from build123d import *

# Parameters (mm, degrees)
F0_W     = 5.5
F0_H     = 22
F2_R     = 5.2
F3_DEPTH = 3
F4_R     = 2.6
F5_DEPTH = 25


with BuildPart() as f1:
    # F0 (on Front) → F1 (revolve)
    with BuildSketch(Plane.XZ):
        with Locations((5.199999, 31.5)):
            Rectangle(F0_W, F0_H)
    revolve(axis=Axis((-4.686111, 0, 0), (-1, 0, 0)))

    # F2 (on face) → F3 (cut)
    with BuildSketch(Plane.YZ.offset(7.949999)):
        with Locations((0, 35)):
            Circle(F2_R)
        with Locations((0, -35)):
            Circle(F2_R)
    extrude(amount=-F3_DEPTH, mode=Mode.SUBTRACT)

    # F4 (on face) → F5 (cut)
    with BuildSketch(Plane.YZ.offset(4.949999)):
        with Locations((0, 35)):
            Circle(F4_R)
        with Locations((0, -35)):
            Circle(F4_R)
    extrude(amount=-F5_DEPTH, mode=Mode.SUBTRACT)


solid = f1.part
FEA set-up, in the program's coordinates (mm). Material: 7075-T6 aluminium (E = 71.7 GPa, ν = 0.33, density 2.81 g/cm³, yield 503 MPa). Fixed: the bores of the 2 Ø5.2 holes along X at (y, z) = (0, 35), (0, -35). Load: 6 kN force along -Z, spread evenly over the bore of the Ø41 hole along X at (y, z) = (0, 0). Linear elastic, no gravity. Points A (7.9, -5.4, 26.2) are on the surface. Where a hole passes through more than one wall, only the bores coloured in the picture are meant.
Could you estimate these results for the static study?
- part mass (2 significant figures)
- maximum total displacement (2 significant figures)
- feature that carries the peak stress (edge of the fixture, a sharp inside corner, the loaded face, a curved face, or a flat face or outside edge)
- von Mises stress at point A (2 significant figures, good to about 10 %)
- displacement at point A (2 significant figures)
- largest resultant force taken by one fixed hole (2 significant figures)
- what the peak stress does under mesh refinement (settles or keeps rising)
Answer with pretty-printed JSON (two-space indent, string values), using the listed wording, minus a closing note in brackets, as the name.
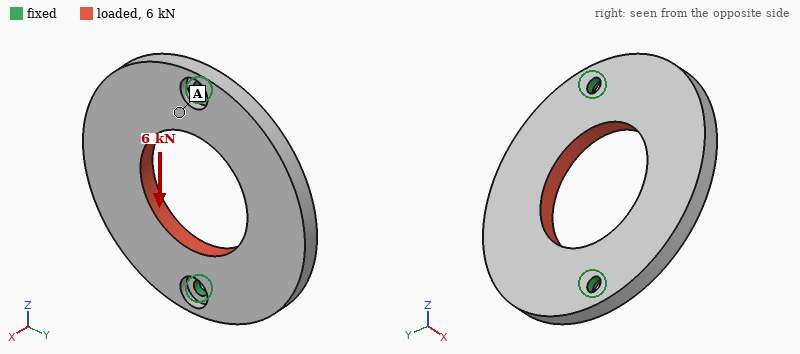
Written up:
{
  "part mass": "66 g",
  "maximum total displacement": "21 µm",
  "feature that carries the peak stress": "edge of the fixture",
  "von Mises stress at point A": "17 MPa",
  "displacement at point A": "13 µm",
  "largest resultant force taken by one fixed hole": "3.0 kN",
  "what the peak stress does under mesh refinement": "keeps rising"
}
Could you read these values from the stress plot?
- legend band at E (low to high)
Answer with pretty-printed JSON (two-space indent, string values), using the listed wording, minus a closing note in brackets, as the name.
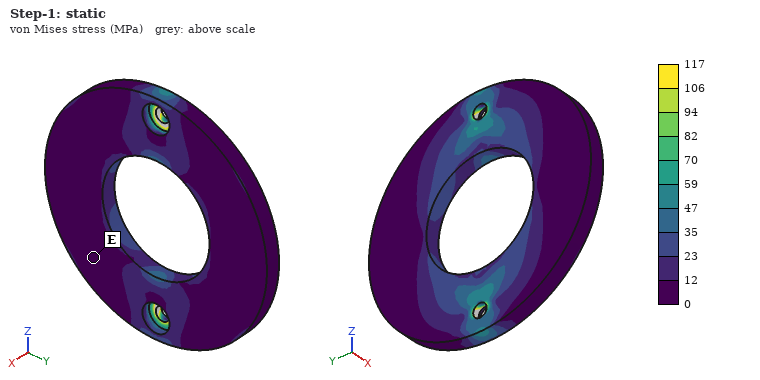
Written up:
{
  "legend band at E": "0 to 12 MPa"
}
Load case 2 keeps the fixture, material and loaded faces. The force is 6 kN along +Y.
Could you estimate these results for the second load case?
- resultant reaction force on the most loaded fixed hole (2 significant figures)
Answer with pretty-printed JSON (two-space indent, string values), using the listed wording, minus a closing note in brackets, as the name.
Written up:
{
  "resultant reaction force on the most loaded fixed hole": "3.0 kN"
}
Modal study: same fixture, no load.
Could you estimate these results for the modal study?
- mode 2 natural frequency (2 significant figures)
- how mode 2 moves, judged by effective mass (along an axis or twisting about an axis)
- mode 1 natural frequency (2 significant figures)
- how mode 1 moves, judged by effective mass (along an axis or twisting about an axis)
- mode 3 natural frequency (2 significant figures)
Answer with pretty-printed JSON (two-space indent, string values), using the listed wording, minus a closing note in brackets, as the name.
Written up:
{
  "mode 2 natural frequency": "2000 Hz",
  "how mode 2 moves, judged by effective mass": "along X",
  "mode 1 natural frequency": "1300 Hz",
  "how mode 1 moves, judged by effective mass": "twisting about Z",
  "mode 3 natural frequency": "4300 Hz"
}
